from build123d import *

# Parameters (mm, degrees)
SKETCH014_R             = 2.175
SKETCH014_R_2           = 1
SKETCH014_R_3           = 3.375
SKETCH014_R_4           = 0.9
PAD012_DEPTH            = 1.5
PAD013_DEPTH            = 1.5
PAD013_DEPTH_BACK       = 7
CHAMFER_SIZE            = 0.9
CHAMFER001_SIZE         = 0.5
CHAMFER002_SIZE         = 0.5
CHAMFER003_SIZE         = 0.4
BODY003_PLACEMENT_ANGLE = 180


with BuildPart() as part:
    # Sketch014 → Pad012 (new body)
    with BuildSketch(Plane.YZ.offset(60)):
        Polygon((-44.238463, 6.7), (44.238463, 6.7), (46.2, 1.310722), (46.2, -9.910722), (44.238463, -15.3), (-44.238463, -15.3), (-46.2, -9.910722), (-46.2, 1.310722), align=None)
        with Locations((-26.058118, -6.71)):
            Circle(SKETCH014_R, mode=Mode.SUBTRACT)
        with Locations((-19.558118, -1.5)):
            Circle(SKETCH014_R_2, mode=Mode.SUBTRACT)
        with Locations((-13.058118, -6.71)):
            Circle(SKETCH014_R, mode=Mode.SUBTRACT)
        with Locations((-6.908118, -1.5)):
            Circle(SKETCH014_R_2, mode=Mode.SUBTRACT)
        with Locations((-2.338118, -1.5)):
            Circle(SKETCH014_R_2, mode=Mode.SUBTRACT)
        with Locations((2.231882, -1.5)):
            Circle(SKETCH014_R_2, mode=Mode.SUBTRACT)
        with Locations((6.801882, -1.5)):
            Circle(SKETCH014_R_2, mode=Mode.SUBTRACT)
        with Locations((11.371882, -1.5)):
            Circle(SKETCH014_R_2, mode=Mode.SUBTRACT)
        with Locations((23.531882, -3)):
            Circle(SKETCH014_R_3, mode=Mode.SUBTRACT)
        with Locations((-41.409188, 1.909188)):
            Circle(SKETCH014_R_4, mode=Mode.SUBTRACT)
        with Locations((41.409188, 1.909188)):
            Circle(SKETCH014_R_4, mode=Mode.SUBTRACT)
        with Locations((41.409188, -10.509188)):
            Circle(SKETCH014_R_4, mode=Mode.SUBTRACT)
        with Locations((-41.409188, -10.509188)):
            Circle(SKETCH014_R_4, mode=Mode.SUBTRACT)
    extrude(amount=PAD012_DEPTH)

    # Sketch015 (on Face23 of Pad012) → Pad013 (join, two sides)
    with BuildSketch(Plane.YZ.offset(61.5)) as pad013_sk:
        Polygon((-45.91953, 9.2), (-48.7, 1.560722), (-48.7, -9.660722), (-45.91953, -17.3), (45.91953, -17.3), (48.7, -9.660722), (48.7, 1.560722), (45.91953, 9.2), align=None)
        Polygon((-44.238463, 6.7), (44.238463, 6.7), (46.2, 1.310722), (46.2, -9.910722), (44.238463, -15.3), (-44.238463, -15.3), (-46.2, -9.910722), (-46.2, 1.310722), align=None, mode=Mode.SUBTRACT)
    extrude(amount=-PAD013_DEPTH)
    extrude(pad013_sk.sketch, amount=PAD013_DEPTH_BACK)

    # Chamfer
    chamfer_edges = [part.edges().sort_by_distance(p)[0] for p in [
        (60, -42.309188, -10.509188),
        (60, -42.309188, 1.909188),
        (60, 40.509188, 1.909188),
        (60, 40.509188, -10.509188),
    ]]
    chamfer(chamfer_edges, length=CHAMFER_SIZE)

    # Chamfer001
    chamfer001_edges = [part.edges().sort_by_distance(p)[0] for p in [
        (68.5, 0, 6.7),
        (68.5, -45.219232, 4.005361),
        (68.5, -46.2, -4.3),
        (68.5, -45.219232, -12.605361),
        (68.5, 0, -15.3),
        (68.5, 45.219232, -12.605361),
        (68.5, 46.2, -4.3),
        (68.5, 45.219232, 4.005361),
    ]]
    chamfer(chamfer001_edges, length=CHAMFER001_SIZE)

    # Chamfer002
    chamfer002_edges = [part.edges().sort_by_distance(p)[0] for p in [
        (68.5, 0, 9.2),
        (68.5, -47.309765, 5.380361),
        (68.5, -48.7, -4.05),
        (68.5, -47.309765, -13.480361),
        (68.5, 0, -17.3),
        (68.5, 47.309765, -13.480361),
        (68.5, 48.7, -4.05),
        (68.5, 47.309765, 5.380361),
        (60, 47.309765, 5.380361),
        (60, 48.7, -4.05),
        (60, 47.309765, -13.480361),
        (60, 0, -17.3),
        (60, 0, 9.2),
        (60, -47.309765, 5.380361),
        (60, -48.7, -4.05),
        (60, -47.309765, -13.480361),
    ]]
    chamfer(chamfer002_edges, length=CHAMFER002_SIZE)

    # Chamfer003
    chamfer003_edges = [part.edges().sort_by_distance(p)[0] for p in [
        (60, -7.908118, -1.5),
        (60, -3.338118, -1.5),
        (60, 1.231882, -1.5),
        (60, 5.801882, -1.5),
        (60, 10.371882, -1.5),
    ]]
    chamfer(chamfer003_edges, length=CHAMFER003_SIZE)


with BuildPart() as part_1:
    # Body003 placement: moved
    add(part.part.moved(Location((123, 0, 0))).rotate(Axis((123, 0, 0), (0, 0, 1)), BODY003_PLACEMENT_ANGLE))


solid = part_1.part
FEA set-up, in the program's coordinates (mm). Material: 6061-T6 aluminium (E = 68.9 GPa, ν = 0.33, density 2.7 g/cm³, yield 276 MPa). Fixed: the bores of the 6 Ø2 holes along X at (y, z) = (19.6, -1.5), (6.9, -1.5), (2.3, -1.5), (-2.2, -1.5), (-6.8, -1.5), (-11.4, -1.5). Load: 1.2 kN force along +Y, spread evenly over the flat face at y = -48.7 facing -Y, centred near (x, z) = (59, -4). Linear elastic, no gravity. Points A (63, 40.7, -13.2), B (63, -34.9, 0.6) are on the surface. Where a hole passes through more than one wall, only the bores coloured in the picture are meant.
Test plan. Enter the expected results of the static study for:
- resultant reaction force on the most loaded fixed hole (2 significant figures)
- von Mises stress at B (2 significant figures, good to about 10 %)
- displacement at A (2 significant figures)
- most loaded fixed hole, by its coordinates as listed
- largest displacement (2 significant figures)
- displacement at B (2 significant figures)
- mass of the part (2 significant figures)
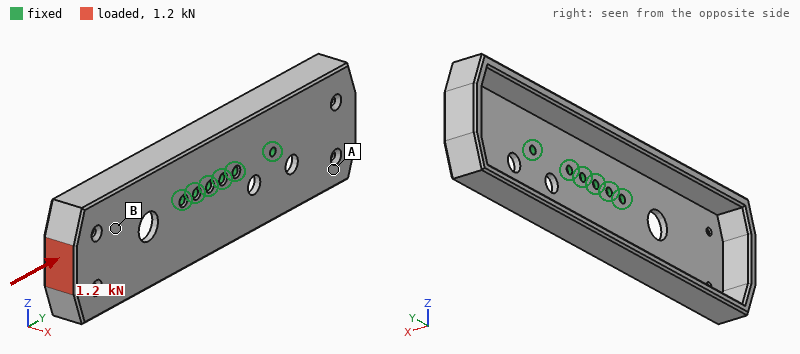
370 N
33 MPa
0.081 mm
(-11.4, -1.5)
0.25 mm
0.11 mm
20 g
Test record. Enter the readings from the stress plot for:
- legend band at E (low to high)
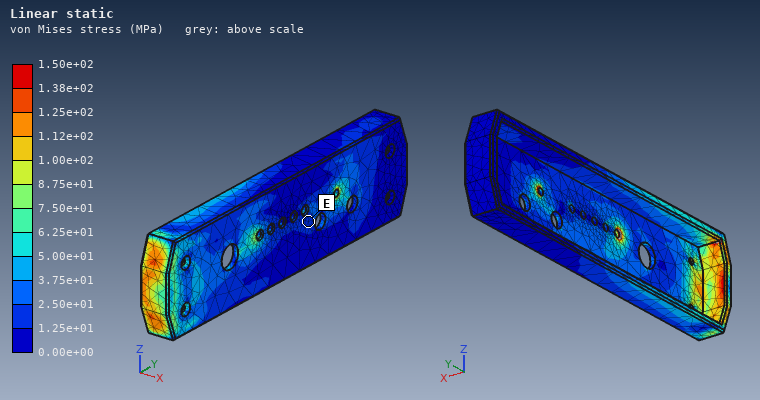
1.25e+01 to 2.50e+01 MPa
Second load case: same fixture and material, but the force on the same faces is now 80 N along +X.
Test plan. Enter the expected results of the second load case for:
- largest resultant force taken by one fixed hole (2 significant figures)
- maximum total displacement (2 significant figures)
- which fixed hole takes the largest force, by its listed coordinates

180 N
0.24 mm
(-11.4, -1.5)
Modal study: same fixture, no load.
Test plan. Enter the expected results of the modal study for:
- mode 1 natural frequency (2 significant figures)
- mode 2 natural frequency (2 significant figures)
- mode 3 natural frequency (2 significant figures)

1500 Hz
1900 Hz
2300 Hz
